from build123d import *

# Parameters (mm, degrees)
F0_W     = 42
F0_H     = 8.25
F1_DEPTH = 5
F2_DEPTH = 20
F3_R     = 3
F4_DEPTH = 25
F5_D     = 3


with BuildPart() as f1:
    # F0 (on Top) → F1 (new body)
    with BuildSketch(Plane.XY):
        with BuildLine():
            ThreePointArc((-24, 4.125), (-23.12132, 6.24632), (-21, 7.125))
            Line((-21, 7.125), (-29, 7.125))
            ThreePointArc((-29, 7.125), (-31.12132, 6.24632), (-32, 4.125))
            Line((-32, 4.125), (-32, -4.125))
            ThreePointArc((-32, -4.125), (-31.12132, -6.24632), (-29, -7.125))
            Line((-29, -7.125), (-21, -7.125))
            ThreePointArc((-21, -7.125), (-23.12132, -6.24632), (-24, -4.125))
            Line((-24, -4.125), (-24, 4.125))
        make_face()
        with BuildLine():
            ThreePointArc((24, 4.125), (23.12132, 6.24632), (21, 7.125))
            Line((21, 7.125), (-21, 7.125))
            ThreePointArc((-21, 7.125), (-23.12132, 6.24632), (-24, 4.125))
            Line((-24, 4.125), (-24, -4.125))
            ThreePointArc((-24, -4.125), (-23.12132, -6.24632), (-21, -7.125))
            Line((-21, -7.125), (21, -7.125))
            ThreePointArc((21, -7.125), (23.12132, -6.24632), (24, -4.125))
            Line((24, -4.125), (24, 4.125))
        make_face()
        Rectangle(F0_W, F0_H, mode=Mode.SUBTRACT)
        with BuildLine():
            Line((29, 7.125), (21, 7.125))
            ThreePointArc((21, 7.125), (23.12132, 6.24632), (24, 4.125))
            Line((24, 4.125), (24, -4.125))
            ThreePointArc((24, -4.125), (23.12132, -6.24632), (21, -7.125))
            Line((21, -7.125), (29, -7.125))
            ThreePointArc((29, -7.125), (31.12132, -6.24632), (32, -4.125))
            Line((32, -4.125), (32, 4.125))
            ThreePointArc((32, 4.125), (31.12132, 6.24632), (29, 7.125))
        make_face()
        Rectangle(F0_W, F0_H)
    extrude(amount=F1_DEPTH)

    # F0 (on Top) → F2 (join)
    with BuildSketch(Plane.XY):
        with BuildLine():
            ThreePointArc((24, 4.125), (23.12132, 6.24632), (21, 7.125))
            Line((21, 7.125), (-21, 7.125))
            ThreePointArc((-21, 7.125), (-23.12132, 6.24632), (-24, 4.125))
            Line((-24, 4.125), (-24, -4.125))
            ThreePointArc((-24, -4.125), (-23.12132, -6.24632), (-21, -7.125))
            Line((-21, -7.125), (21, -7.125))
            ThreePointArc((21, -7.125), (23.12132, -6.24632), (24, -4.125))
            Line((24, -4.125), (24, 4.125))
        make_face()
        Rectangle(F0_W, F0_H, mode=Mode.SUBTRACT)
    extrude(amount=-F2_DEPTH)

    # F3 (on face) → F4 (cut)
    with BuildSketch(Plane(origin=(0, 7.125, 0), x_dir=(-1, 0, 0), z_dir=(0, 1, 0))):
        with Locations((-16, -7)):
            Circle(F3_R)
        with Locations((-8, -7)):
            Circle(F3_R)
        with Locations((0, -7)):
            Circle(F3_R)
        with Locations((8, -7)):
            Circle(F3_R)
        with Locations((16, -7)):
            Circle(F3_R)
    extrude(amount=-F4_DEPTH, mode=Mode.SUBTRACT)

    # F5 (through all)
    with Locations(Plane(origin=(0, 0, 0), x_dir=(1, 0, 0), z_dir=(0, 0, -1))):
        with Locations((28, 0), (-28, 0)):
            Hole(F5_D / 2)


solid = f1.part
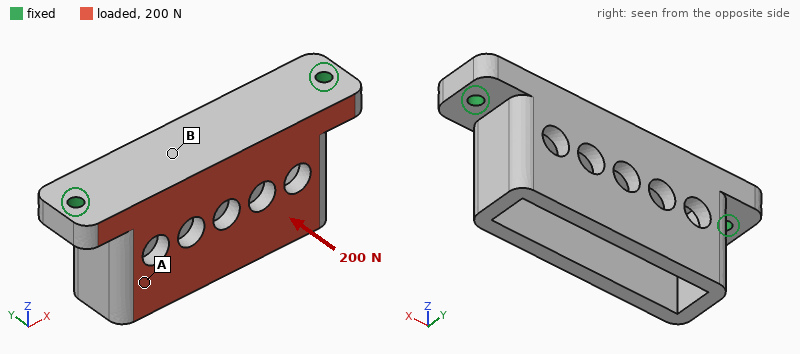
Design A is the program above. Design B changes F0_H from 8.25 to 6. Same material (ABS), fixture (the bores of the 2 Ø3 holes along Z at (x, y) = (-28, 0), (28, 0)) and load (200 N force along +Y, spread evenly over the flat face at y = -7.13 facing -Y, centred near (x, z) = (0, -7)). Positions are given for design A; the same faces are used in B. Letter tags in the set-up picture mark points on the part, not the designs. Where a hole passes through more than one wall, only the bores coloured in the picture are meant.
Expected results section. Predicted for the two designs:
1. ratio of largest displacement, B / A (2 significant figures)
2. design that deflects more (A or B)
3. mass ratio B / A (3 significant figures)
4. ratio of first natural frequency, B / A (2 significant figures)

0.73
A
1.15
0.93
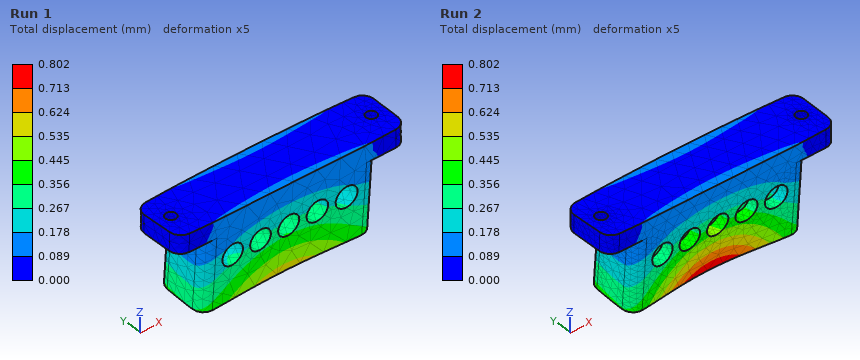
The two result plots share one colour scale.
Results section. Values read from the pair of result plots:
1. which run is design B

Run 1
